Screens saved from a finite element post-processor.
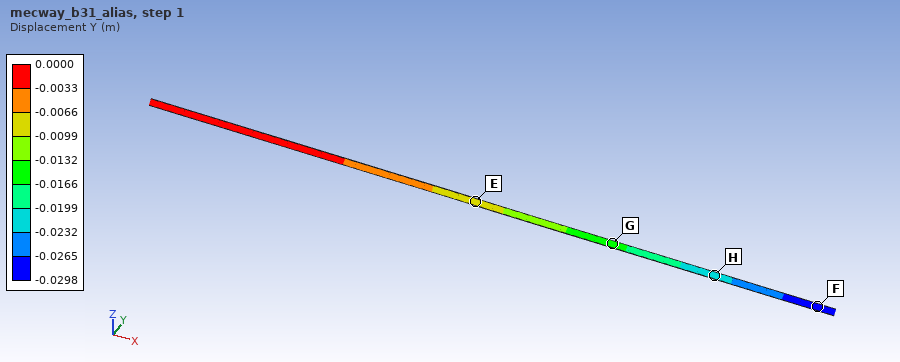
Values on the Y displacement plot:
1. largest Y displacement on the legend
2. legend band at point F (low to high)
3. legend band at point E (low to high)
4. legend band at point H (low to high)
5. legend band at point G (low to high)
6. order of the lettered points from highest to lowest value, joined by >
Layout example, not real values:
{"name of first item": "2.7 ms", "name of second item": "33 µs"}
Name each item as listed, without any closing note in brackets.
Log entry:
{"largest Y displacement on the legend": "0.0000 m", "legend band at point F": "-0.0298 to -0.0265 m", "legend band at point E": "-0.0099 to -0.0066 m", "legend band at point H": "-0.0232 to -0.0199 m", "legend band at point G": "-0.0166 to -0.0132 m", "order of the lettered points from highest to lowest value, joined by >": "E > G > H > F"}
